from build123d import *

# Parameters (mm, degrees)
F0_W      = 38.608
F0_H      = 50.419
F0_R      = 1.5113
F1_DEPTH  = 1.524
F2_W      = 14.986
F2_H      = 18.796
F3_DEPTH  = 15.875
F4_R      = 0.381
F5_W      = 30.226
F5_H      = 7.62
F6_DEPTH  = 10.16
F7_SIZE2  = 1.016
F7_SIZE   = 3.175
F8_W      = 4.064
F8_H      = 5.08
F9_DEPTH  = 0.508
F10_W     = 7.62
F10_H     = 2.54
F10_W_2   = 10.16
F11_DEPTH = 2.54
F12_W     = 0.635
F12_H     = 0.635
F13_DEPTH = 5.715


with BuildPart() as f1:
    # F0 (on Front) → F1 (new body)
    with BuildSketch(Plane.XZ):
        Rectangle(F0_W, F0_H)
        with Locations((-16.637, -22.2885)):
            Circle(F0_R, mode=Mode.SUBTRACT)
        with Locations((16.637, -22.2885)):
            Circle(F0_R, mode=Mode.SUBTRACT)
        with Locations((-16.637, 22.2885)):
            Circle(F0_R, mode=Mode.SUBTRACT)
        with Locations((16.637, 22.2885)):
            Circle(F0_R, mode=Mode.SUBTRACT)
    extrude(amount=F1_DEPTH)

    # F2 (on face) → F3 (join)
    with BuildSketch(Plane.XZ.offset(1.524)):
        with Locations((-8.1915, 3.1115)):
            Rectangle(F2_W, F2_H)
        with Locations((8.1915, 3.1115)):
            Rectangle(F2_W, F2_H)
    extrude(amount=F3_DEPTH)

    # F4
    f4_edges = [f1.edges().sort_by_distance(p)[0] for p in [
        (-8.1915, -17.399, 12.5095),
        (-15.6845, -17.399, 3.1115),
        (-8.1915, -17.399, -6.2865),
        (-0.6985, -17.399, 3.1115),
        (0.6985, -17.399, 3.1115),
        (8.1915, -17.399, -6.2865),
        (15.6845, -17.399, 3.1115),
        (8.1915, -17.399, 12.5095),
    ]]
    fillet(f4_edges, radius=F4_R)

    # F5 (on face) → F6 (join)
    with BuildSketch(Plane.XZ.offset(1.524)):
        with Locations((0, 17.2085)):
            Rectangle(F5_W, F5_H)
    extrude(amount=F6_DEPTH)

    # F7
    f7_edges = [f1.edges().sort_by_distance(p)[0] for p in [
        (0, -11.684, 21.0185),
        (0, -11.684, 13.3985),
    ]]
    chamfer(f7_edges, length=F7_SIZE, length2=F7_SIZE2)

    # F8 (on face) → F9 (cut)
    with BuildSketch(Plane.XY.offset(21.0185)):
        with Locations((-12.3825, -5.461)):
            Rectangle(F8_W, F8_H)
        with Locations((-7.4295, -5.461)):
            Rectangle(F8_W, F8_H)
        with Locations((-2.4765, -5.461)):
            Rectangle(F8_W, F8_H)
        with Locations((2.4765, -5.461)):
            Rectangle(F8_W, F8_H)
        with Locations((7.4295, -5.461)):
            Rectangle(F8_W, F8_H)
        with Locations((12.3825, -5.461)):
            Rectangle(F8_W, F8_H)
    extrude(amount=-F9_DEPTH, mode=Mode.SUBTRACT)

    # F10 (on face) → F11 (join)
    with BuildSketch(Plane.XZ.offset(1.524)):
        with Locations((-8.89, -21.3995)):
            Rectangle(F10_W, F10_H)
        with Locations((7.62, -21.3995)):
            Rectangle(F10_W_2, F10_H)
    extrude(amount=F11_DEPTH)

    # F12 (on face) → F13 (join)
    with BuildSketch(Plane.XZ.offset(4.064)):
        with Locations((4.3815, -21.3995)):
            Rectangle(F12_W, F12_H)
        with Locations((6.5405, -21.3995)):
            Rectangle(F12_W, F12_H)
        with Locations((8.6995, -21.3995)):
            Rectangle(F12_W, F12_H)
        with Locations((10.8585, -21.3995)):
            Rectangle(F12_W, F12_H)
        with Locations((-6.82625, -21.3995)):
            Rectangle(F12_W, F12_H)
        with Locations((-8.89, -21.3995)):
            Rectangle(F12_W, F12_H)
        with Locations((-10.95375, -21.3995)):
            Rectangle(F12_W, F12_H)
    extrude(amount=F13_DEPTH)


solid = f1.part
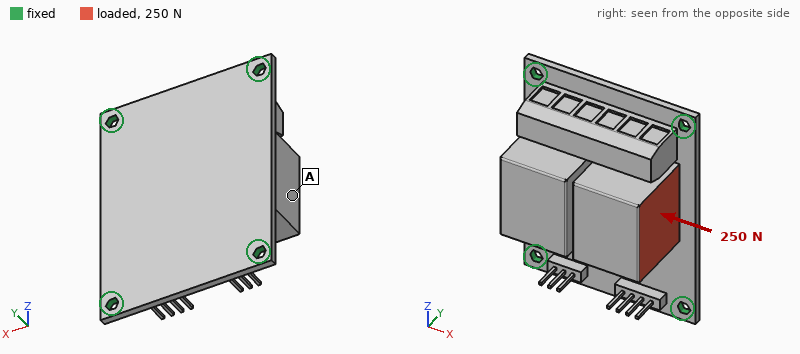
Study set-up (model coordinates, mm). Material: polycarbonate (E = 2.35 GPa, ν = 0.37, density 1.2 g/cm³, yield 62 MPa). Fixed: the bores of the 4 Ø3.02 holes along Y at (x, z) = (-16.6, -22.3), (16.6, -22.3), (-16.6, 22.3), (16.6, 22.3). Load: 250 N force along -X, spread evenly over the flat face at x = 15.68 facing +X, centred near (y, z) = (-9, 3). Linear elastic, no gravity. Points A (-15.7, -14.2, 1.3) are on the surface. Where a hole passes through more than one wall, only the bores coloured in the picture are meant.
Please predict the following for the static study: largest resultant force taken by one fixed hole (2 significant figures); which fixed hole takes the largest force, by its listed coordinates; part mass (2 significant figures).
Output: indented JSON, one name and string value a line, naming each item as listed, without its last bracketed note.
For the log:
{
  "largest resultant force taken by one fixed hole": "140 N",
  "which fixed hole takes the largest force, by its listed coordinates": "(-16.6, 22.3)",
  "part mass": "17 g"
}
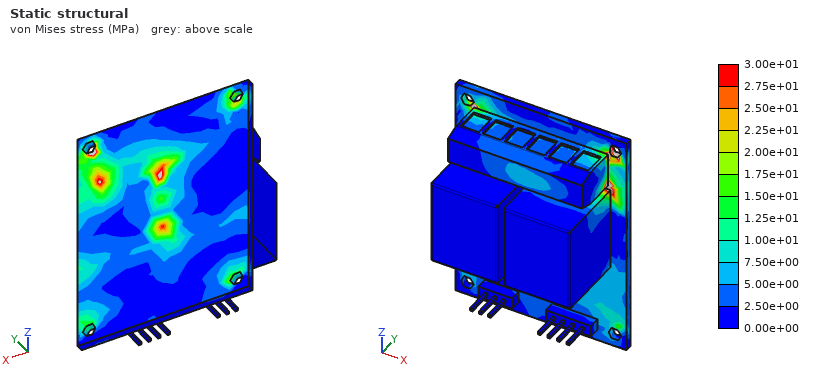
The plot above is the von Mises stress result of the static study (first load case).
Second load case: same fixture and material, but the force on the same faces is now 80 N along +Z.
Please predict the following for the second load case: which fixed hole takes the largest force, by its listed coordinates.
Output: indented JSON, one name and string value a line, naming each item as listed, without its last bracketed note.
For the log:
{
  "which fixed hole takes the largest force, by its listed coordinates": "(16.6, 22.3)"
}
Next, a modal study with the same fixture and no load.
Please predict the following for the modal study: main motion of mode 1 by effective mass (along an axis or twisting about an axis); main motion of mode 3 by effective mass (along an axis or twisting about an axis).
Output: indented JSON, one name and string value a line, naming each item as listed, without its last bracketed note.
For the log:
{
  "main motion of mode 1 by effective mass": "along Y",
  "main motion of mode 3 by effective mass": "along X"
}
